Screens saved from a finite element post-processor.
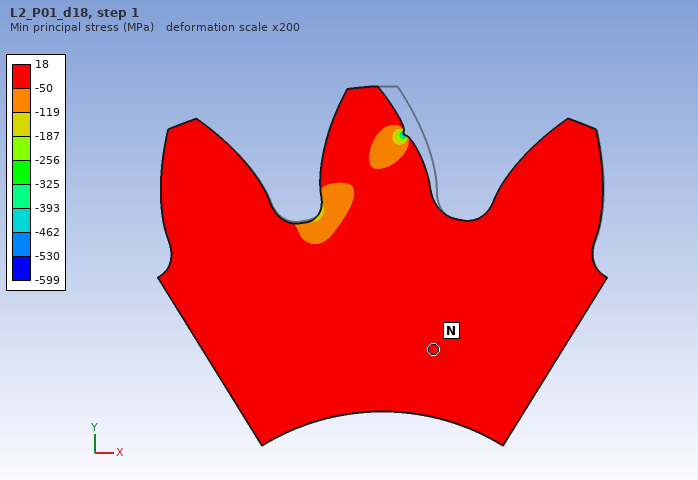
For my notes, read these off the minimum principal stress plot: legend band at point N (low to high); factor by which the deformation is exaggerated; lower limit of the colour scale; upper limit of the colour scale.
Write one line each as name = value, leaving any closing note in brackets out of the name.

legend band at point N = -50 to 18 MPa
factor by which the deformation is exaggerated = 200
lower limit of the colour scale = -599 MPa
upper limit of the colour scale = 18 MPa
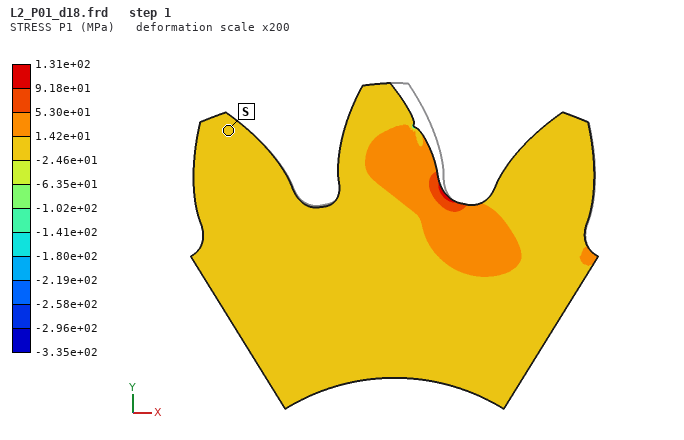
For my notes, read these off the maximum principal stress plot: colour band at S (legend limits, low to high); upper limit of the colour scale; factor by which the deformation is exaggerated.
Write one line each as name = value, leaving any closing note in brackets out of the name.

colour band at S = -2.46e+01 to 1.42e+01 MPa
upper limit of the colour scale = 1.31e+02 MPa
factor by which the deformation is exaggerated = 200
